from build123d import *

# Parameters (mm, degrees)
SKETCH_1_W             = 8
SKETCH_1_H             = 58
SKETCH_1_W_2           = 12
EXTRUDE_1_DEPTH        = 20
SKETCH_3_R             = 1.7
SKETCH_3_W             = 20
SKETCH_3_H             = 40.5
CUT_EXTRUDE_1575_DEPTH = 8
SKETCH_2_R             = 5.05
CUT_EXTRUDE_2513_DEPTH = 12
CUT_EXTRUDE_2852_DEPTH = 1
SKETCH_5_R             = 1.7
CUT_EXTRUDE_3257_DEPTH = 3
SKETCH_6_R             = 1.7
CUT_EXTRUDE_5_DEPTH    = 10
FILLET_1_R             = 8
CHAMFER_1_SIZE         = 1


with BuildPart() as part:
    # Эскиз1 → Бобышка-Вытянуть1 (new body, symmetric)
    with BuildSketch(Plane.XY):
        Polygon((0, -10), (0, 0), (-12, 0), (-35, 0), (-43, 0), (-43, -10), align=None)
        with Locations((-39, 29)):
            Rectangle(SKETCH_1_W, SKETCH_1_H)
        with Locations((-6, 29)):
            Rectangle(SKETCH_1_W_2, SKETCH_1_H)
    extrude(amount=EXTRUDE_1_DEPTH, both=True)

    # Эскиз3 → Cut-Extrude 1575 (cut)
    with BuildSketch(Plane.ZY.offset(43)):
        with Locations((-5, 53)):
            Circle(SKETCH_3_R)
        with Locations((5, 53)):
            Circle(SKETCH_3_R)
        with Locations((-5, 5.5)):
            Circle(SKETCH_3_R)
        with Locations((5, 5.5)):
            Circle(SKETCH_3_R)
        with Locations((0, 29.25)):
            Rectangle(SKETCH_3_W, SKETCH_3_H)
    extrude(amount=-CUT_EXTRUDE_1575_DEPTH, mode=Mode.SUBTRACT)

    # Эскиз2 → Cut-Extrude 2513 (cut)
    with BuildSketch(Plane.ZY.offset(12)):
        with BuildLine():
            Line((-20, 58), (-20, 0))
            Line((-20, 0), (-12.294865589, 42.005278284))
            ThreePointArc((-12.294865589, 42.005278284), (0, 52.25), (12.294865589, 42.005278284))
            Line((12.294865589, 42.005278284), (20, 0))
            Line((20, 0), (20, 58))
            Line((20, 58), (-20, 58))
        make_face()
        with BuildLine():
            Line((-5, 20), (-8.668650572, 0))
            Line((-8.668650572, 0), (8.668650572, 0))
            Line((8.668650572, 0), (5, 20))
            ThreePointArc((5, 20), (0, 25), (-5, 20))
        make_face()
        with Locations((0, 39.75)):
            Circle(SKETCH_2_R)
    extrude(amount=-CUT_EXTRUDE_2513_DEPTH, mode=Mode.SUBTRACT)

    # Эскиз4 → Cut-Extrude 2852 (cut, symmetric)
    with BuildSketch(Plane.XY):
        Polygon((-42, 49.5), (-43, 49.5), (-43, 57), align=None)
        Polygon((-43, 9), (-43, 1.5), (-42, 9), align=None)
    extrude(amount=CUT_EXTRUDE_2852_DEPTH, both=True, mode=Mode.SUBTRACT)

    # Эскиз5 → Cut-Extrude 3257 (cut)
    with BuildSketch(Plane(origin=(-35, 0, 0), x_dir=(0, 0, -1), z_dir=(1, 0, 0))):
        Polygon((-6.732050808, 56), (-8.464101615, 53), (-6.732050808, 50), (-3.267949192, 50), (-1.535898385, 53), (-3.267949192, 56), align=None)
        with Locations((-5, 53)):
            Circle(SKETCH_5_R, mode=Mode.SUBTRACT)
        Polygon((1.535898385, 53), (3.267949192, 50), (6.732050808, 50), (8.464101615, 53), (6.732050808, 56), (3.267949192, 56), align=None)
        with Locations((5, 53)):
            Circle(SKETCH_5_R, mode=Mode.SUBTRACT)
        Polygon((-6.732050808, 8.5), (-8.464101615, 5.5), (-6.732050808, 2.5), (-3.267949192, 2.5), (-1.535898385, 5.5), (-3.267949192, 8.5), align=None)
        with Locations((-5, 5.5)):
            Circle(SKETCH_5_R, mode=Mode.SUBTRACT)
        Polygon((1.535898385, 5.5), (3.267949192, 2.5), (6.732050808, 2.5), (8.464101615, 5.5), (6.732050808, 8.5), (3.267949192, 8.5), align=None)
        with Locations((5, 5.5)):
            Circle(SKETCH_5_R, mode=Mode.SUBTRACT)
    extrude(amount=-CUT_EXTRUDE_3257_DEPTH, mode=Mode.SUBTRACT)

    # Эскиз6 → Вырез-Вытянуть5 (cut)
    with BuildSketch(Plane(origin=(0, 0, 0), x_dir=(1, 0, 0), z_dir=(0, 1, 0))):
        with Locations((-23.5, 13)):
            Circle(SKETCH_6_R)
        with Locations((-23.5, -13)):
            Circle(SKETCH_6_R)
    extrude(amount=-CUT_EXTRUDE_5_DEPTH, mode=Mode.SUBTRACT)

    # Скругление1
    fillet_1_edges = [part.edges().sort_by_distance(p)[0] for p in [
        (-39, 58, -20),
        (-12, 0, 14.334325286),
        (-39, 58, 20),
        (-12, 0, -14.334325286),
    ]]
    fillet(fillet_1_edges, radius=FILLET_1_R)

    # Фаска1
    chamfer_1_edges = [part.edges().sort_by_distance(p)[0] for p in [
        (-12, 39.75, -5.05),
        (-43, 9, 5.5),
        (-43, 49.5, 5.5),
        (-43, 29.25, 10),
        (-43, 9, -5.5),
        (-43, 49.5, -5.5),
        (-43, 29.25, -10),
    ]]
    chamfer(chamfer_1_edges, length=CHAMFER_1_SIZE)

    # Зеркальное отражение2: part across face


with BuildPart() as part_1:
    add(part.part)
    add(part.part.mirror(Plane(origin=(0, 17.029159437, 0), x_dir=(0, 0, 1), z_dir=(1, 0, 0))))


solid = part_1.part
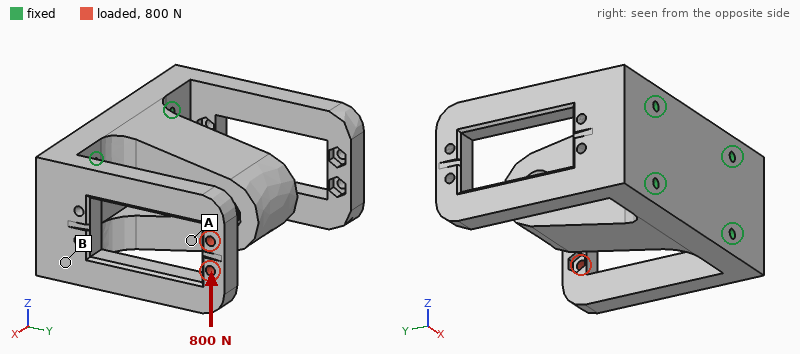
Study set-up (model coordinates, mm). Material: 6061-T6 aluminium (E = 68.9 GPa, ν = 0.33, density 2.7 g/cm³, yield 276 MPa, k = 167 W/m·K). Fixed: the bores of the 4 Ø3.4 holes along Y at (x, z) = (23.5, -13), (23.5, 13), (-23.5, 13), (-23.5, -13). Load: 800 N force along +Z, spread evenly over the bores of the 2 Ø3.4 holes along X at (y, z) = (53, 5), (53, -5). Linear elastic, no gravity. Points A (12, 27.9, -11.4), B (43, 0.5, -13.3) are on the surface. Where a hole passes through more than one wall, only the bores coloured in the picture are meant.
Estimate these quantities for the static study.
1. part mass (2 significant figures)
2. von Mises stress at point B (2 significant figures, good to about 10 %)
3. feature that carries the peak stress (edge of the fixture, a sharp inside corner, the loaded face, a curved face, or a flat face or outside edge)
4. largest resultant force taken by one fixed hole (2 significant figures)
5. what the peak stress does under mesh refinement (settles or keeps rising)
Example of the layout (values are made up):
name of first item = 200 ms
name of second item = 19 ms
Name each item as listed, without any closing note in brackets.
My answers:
part mass = 230 g
von Mises stress at point B = 25 MPa
feature that carries the peak stress = edge of the fixture
largest resultant force taken by one fixed hole = 1.6 kN
what the peak stress does under mesh refinement = keeps rising
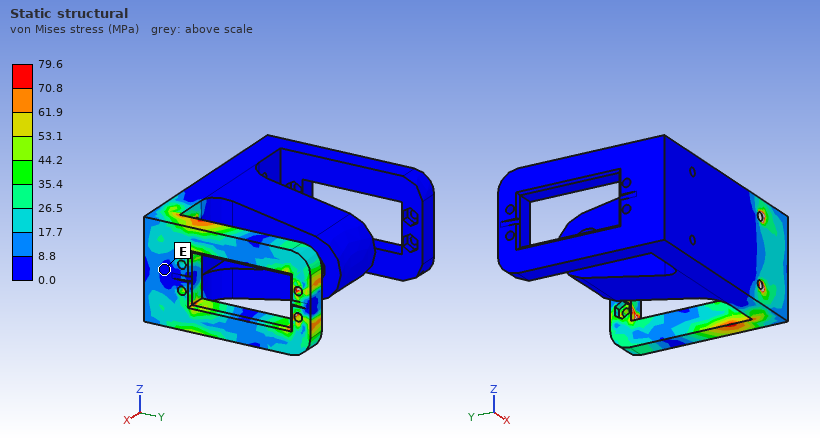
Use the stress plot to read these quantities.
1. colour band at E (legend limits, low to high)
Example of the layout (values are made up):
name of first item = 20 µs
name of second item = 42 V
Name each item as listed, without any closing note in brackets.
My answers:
colour band at E = 0.0 to 8.8 MPa
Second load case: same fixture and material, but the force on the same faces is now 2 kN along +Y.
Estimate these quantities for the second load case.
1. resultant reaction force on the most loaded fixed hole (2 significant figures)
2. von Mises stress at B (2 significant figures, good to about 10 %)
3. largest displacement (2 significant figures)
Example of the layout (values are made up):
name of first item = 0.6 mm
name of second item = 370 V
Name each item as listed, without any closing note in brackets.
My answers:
resultant reaction force on the most loaded fixed hole = 1.1 kN
von Mises stress at B = 19 MPa
largest displacement = 0.20 mm
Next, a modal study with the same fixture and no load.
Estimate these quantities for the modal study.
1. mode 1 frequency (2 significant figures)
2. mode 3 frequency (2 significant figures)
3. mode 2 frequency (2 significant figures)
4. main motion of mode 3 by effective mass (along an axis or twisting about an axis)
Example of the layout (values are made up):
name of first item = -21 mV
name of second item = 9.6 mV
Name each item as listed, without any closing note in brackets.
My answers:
mode 1 frequency = 1400 Hz
mode 3 frequency = 2700 Hz
mode 2 frequency = 1400 Hz
main motion of mode 3 by effective mass = along Z
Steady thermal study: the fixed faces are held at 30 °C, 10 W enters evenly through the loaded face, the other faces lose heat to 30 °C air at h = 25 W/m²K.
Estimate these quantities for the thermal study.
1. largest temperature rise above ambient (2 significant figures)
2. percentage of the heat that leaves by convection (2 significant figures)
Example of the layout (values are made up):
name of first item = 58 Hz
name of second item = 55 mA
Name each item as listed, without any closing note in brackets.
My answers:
largest temperature rise above ambient = 24 K
percentage of the heat that leaves by convection = 17 %
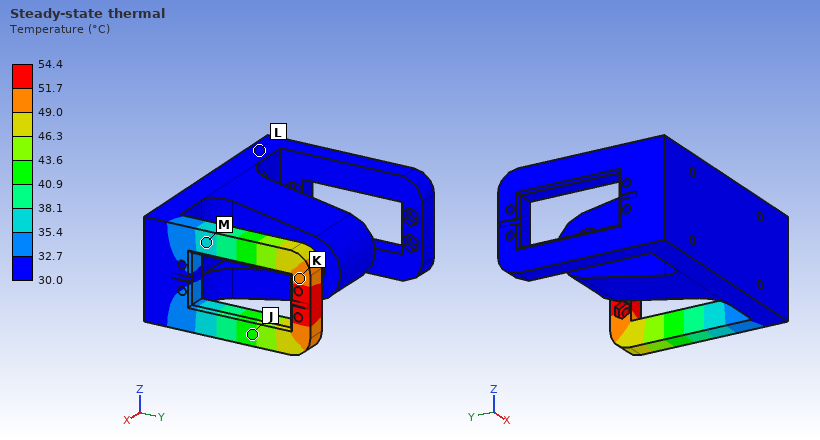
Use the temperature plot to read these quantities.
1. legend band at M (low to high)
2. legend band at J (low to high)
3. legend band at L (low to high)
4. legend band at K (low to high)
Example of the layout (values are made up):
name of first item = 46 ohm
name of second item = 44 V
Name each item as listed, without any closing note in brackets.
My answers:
legend band at M = 35.4 to 38.1 °C
legend band at J = 40.9 to 43.6 °C
legend band at L = 30.0 to 32.7 °C
legend band at K = 49.0 to 51.7 °C
